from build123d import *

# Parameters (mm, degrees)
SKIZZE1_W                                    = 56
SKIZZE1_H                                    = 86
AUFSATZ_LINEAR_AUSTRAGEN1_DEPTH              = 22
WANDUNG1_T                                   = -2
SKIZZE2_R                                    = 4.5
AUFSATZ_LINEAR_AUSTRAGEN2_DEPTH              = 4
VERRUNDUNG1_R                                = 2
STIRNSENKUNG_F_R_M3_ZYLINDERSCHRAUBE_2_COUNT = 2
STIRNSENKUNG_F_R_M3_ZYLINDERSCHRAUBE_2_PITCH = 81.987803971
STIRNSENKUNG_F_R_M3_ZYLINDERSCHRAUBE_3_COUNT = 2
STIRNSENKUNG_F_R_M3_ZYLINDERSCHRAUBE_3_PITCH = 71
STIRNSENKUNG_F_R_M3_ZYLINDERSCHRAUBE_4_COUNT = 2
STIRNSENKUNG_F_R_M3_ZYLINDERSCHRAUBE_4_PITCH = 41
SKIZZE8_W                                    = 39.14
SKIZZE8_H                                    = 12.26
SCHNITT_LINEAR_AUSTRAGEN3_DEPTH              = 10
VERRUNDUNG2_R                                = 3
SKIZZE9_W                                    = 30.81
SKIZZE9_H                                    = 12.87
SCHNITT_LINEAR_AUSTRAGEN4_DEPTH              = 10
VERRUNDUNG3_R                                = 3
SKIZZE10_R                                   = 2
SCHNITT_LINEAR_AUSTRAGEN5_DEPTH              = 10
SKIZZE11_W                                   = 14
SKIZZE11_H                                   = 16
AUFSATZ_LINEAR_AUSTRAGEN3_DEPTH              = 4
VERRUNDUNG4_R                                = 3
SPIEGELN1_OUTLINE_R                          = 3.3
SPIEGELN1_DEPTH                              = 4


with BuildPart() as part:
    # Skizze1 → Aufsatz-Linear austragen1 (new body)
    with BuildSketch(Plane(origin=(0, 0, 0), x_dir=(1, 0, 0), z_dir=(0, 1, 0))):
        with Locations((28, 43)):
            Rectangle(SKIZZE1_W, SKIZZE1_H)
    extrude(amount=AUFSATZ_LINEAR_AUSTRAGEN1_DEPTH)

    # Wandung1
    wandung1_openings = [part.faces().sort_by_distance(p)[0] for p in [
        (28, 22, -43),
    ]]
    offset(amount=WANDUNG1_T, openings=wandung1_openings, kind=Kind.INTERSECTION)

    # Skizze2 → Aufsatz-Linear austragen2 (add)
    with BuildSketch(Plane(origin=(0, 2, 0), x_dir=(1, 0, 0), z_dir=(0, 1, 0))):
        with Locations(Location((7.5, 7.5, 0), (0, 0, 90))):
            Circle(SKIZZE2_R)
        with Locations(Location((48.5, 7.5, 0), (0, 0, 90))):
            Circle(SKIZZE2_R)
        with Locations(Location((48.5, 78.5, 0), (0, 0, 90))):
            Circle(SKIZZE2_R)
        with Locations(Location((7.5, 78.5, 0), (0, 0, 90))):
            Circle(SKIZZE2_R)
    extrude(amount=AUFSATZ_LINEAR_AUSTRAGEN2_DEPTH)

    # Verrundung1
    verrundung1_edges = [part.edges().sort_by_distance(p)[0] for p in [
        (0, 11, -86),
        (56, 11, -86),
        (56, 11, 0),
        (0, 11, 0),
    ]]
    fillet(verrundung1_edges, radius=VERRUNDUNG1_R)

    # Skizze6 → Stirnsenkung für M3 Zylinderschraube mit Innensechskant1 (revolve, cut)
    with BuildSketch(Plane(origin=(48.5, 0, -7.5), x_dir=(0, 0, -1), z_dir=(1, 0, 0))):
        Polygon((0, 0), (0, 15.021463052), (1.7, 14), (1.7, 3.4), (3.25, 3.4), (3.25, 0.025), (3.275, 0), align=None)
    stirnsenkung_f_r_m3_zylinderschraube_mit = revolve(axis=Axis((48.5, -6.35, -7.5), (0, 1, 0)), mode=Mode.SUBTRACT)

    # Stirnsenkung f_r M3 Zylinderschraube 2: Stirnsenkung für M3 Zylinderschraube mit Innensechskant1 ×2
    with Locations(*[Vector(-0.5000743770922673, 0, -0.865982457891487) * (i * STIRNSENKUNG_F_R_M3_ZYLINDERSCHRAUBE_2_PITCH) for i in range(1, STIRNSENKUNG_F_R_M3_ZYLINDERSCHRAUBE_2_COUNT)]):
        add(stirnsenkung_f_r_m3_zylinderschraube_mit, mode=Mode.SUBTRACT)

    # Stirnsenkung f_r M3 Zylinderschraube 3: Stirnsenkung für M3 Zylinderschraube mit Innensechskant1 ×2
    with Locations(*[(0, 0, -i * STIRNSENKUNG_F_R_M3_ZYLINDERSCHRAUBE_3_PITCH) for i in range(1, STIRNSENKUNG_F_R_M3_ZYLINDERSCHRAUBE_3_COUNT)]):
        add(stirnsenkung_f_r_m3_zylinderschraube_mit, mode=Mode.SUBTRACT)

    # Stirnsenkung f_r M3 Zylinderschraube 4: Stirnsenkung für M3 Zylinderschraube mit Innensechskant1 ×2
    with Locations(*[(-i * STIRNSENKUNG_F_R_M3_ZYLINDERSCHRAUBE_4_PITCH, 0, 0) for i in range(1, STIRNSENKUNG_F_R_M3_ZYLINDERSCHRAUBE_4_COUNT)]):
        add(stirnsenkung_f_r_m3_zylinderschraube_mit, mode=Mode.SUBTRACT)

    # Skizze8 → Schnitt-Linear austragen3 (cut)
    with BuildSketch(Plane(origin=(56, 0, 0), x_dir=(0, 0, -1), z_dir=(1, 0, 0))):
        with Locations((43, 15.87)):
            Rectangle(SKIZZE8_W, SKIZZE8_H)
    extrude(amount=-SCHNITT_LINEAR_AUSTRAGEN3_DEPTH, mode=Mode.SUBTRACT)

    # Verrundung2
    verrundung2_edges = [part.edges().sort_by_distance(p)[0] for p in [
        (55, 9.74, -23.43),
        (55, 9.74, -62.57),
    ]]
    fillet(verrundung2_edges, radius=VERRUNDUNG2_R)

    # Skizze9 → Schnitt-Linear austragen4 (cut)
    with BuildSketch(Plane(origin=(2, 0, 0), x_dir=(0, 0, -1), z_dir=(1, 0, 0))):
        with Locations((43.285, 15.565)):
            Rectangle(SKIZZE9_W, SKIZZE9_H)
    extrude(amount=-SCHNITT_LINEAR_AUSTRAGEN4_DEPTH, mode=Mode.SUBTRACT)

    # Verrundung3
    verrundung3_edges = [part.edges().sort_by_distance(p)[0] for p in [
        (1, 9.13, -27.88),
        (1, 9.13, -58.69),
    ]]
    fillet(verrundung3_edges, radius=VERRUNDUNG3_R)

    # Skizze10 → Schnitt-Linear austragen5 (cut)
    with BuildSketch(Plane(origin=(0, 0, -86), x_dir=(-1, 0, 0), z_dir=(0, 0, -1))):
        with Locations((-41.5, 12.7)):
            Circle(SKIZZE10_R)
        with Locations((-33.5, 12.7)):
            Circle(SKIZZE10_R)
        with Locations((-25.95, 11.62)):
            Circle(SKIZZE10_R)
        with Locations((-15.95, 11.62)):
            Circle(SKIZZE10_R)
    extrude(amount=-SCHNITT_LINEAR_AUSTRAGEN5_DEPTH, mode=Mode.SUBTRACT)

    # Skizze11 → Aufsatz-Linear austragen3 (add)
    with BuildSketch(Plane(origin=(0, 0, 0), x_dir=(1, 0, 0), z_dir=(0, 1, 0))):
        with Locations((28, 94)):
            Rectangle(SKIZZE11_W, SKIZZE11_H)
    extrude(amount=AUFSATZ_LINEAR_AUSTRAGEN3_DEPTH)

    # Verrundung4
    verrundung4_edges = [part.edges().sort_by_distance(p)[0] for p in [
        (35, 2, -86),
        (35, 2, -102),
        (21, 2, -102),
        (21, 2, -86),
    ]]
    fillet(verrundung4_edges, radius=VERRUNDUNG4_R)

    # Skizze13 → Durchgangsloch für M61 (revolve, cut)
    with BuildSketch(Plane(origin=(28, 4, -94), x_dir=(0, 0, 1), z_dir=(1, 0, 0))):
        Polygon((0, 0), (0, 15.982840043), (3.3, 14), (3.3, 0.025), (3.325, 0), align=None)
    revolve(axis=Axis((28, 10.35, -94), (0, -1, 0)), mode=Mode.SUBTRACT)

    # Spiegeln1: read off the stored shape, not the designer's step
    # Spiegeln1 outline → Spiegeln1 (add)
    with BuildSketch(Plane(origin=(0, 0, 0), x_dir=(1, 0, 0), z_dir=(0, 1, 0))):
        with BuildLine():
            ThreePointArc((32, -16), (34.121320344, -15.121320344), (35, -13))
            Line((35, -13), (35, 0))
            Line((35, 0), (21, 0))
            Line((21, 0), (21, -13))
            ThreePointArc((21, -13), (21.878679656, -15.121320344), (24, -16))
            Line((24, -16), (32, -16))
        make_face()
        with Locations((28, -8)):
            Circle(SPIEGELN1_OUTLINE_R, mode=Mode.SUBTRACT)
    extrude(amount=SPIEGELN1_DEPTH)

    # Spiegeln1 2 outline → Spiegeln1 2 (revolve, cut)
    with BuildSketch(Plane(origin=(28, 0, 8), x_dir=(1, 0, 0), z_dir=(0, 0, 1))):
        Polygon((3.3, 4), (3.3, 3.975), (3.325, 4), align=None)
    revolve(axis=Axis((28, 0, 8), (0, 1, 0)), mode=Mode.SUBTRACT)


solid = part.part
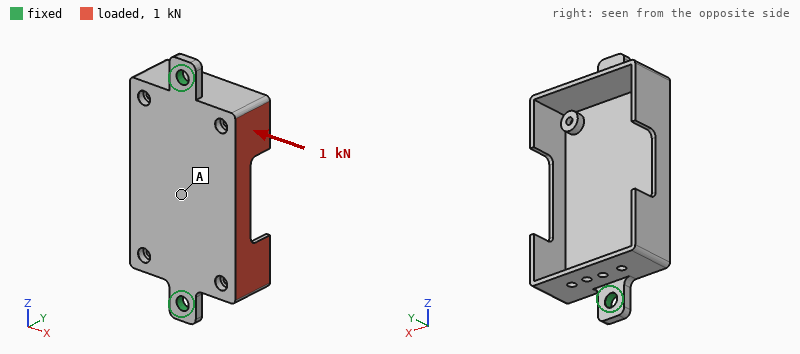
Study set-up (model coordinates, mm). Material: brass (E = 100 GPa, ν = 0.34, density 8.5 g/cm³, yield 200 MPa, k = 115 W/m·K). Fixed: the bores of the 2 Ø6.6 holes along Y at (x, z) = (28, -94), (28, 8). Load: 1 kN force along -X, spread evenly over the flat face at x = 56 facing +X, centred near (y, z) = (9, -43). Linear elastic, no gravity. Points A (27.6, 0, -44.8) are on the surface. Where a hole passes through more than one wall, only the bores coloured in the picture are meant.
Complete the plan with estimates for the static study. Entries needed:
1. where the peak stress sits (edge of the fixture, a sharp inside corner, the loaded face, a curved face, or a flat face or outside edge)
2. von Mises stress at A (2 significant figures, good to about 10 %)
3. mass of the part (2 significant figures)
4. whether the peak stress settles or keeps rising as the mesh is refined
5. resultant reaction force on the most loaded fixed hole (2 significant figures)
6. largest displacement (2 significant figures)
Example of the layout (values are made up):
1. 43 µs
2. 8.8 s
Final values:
1. edge of the fixture
2. 9.0 MPa
3. 180 g
4. keeps rising
5. 510 N
6. 0.23 mm
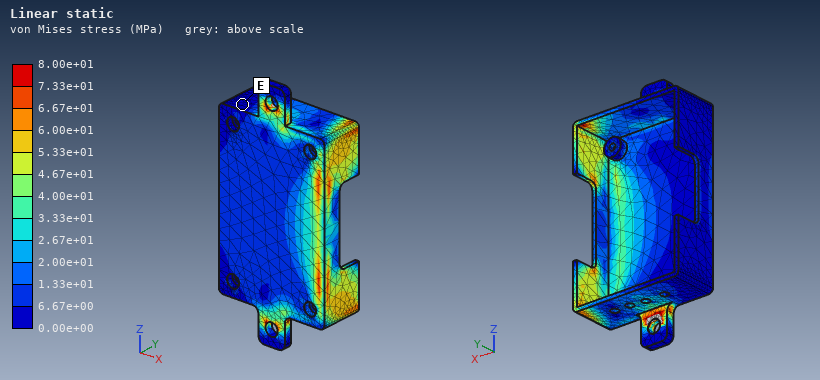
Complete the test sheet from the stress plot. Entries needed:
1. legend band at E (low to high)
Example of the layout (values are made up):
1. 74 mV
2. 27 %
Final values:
1. 0.00e+00 to 6.67e+00 MPa
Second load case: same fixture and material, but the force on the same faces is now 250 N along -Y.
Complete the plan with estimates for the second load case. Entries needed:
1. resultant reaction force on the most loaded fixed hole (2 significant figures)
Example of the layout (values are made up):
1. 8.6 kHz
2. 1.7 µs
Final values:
1. 130 N
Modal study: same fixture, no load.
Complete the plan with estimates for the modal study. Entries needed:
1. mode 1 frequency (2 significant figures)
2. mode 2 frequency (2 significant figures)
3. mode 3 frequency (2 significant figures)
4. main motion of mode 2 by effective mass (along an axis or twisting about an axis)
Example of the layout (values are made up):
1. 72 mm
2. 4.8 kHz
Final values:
1. 1000 Hz
2. 1400 Hz
3. 1600 Hz
4. along Y
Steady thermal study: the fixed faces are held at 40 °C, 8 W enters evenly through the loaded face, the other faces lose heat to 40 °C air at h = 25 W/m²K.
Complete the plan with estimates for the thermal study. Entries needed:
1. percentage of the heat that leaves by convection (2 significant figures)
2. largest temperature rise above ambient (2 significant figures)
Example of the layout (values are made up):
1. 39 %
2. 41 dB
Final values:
1. 36 %
2. 14 K
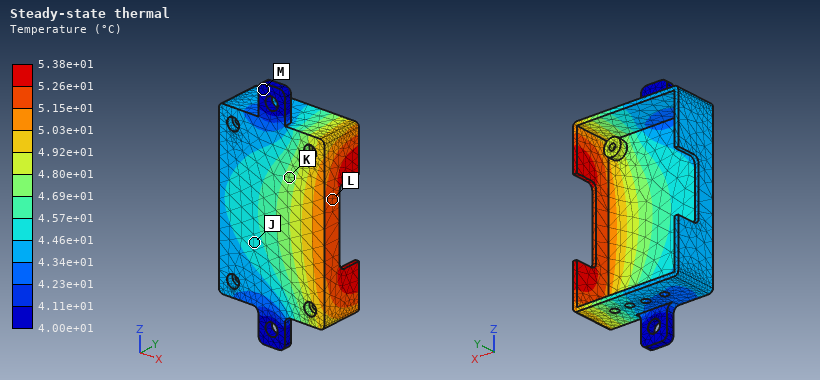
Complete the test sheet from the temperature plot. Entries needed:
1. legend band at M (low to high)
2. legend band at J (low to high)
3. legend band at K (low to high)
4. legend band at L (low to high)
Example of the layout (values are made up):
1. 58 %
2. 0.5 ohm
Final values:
1. 4.00e+01 to 4.11e+01 °C
2. 4.46e+01 to 4.57e+01 °C
3. 4.69e+01 to 4.80e+01 °C
4. 5.15e+01 to 5.26e+01 °C
